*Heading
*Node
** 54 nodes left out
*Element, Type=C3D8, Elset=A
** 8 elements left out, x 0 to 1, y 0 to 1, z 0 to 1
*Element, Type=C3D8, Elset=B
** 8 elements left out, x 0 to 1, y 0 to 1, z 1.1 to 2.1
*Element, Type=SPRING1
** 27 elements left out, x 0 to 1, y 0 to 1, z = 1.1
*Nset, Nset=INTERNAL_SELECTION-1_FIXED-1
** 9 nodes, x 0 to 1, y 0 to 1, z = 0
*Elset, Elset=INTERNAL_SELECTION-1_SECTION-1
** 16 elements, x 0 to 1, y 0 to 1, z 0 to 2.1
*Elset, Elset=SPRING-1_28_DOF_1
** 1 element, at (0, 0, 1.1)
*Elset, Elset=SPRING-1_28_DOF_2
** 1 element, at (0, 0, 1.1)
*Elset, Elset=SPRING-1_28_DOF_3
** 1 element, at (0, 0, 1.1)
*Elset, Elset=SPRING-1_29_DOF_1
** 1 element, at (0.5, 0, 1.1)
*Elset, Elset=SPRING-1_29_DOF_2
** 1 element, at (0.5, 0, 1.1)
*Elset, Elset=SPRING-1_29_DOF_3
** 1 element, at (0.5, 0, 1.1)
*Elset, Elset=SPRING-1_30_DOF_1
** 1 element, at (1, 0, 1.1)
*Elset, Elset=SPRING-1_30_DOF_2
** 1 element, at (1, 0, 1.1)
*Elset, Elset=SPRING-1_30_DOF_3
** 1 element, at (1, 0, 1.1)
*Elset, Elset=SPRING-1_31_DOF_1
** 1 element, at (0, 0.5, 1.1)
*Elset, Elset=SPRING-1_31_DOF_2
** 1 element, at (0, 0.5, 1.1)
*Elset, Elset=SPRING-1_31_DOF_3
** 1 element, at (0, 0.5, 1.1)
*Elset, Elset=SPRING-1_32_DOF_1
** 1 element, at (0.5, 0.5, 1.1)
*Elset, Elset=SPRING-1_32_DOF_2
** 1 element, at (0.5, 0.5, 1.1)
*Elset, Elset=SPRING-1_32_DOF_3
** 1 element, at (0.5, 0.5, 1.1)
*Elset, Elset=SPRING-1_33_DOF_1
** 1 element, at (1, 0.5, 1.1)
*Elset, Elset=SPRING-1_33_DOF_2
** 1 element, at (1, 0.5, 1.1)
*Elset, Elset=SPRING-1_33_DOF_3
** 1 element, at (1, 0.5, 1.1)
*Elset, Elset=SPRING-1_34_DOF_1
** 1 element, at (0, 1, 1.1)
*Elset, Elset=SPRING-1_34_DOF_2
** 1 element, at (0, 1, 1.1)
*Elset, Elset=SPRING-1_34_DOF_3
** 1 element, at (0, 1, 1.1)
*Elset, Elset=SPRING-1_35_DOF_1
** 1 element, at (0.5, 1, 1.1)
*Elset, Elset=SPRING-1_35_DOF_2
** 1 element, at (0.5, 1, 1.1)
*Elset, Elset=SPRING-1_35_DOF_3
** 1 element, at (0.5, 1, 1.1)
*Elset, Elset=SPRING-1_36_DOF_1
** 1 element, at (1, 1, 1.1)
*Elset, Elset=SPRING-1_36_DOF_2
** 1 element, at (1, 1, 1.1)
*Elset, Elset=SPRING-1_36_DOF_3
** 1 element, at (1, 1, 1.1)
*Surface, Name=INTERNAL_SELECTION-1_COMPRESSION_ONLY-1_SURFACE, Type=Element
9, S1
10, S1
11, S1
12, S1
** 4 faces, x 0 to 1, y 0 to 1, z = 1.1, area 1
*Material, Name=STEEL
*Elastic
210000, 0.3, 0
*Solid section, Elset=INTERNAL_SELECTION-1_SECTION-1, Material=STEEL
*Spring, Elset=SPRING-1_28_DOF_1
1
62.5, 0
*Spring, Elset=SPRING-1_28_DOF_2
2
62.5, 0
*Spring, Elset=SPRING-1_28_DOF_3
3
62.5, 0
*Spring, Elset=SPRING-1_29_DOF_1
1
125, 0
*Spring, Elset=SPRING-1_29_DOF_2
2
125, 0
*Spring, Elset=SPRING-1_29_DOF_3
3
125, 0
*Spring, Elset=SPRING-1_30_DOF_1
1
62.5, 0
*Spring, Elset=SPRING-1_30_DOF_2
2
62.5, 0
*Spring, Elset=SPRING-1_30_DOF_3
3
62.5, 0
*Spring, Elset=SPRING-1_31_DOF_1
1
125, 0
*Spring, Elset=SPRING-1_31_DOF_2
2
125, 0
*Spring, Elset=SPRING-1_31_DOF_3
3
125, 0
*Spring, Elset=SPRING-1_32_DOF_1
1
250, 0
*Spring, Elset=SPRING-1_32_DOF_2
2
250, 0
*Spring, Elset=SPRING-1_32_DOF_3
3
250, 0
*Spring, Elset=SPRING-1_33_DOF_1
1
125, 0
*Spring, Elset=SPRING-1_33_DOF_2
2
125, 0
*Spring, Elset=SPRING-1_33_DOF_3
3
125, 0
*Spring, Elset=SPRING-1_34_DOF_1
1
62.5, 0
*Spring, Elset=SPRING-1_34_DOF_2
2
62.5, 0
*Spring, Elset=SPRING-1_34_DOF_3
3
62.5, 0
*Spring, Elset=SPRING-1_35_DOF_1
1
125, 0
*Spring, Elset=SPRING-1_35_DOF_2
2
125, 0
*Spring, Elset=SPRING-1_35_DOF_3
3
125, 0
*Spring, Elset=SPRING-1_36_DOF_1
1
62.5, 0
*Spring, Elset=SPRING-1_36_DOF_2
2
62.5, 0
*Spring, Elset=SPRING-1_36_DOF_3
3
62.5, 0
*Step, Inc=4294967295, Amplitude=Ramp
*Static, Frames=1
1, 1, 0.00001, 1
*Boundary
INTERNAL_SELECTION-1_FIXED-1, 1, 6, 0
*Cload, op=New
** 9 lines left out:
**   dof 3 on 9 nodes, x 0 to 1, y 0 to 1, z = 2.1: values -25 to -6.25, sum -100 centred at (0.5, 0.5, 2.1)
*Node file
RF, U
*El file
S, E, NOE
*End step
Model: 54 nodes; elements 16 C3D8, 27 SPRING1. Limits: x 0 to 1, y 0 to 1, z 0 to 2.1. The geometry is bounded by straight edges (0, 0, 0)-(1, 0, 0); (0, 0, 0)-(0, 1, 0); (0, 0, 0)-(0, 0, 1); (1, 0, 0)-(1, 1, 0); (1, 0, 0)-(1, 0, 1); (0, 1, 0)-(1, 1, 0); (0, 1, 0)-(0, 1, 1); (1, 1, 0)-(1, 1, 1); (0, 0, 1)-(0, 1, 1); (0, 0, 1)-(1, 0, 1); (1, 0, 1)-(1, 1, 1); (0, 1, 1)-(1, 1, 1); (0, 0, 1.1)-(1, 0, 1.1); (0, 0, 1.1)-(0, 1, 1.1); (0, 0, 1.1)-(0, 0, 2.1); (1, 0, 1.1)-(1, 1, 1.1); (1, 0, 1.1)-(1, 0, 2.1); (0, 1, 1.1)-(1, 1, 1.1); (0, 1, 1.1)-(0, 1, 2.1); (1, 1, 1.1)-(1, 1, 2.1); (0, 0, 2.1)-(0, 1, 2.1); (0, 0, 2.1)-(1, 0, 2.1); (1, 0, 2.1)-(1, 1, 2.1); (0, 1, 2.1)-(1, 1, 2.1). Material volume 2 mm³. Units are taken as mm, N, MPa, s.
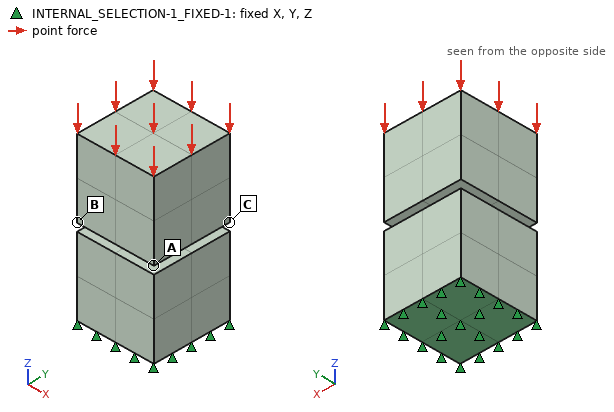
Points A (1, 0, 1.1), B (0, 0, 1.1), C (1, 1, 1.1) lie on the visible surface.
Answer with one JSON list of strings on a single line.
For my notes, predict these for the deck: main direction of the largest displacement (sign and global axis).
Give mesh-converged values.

["-Z"]
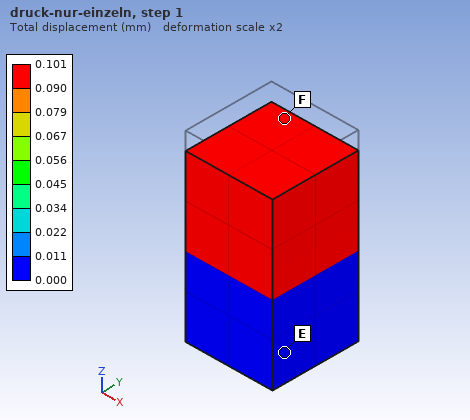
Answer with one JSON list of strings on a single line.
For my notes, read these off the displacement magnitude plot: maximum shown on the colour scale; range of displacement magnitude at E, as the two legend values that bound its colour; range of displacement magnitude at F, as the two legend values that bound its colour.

["0.101 mm", "0.000 to 0.011 mm", "0.090 to 0.101 mm"]
